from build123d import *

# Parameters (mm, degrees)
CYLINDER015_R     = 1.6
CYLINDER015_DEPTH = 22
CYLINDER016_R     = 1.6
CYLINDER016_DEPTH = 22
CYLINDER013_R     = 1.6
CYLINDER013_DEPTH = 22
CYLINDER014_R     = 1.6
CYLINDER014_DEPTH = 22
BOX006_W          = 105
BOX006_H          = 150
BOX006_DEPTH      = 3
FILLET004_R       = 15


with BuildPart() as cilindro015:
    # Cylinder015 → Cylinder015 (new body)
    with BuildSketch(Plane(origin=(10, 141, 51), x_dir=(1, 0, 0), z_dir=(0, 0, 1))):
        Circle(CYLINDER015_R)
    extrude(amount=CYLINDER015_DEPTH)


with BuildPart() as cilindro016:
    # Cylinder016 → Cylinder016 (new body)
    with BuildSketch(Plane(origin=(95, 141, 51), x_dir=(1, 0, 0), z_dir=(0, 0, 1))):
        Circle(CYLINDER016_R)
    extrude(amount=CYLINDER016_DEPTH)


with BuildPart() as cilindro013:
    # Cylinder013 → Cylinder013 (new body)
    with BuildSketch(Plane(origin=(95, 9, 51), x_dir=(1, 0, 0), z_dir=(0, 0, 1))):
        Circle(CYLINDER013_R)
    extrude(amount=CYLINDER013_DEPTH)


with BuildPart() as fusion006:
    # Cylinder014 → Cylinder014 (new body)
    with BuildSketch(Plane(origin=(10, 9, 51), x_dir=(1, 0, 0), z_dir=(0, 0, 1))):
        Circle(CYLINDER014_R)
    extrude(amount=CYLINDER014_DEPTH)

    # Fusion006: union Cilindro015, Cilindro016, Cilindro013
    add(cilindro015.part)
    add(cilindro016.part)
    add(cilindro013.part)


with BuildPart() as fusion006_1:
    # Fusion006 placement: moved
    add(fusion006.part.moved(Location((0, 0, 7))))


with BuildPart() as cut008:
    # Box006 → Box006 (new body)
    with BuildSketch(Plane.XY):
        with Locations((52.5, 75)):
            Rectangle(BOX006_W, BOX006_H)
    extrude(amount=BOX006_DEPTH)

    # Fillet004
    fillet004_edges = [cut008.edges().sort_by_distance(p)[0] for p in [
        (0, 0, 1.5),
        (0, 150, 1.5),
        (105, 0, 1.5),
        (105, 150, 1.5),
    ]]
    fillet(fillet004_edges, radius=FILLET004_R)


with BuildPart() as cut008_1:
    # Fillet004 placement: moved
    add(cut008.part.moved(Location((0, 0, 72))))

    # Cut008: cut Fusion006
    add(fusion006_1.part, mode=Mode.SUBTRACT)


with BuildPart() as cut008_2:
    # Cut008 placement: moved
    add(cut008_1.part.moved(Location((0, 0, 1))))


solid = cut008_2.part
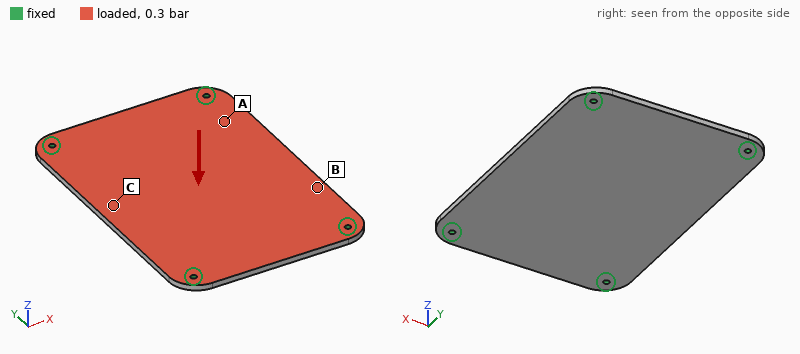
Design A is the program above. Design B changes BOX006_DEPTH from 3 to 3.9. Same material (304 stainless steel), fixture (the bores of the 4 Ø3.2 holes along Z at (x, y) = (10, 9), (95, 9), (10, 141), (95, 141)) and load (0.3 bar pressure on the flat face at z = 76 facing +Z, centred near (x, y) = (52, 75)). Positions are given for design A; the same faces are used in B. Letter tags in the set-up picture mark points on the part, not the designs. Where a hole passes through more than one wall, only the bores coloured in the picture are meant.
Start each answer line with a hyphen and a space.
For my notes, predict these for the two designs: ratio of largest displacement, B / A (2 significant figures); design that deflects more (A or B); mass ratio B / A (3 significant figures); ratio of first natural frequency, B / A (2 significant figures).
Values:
- 0.47
- A
- 1.30
- 1.3
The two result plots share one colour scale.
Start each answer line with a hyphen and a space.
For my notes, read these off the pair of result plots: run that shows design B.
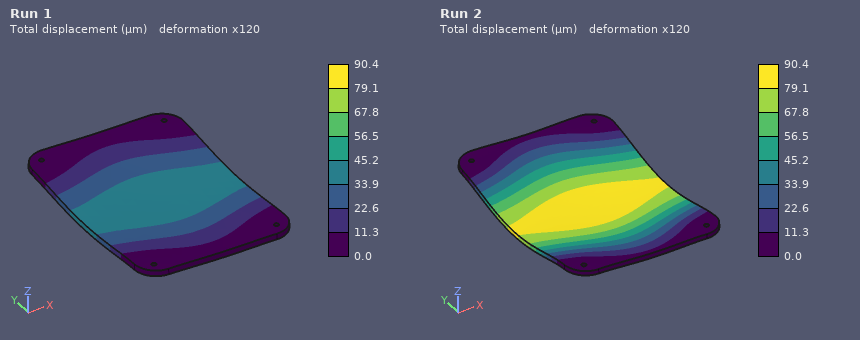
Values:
- Run 1
